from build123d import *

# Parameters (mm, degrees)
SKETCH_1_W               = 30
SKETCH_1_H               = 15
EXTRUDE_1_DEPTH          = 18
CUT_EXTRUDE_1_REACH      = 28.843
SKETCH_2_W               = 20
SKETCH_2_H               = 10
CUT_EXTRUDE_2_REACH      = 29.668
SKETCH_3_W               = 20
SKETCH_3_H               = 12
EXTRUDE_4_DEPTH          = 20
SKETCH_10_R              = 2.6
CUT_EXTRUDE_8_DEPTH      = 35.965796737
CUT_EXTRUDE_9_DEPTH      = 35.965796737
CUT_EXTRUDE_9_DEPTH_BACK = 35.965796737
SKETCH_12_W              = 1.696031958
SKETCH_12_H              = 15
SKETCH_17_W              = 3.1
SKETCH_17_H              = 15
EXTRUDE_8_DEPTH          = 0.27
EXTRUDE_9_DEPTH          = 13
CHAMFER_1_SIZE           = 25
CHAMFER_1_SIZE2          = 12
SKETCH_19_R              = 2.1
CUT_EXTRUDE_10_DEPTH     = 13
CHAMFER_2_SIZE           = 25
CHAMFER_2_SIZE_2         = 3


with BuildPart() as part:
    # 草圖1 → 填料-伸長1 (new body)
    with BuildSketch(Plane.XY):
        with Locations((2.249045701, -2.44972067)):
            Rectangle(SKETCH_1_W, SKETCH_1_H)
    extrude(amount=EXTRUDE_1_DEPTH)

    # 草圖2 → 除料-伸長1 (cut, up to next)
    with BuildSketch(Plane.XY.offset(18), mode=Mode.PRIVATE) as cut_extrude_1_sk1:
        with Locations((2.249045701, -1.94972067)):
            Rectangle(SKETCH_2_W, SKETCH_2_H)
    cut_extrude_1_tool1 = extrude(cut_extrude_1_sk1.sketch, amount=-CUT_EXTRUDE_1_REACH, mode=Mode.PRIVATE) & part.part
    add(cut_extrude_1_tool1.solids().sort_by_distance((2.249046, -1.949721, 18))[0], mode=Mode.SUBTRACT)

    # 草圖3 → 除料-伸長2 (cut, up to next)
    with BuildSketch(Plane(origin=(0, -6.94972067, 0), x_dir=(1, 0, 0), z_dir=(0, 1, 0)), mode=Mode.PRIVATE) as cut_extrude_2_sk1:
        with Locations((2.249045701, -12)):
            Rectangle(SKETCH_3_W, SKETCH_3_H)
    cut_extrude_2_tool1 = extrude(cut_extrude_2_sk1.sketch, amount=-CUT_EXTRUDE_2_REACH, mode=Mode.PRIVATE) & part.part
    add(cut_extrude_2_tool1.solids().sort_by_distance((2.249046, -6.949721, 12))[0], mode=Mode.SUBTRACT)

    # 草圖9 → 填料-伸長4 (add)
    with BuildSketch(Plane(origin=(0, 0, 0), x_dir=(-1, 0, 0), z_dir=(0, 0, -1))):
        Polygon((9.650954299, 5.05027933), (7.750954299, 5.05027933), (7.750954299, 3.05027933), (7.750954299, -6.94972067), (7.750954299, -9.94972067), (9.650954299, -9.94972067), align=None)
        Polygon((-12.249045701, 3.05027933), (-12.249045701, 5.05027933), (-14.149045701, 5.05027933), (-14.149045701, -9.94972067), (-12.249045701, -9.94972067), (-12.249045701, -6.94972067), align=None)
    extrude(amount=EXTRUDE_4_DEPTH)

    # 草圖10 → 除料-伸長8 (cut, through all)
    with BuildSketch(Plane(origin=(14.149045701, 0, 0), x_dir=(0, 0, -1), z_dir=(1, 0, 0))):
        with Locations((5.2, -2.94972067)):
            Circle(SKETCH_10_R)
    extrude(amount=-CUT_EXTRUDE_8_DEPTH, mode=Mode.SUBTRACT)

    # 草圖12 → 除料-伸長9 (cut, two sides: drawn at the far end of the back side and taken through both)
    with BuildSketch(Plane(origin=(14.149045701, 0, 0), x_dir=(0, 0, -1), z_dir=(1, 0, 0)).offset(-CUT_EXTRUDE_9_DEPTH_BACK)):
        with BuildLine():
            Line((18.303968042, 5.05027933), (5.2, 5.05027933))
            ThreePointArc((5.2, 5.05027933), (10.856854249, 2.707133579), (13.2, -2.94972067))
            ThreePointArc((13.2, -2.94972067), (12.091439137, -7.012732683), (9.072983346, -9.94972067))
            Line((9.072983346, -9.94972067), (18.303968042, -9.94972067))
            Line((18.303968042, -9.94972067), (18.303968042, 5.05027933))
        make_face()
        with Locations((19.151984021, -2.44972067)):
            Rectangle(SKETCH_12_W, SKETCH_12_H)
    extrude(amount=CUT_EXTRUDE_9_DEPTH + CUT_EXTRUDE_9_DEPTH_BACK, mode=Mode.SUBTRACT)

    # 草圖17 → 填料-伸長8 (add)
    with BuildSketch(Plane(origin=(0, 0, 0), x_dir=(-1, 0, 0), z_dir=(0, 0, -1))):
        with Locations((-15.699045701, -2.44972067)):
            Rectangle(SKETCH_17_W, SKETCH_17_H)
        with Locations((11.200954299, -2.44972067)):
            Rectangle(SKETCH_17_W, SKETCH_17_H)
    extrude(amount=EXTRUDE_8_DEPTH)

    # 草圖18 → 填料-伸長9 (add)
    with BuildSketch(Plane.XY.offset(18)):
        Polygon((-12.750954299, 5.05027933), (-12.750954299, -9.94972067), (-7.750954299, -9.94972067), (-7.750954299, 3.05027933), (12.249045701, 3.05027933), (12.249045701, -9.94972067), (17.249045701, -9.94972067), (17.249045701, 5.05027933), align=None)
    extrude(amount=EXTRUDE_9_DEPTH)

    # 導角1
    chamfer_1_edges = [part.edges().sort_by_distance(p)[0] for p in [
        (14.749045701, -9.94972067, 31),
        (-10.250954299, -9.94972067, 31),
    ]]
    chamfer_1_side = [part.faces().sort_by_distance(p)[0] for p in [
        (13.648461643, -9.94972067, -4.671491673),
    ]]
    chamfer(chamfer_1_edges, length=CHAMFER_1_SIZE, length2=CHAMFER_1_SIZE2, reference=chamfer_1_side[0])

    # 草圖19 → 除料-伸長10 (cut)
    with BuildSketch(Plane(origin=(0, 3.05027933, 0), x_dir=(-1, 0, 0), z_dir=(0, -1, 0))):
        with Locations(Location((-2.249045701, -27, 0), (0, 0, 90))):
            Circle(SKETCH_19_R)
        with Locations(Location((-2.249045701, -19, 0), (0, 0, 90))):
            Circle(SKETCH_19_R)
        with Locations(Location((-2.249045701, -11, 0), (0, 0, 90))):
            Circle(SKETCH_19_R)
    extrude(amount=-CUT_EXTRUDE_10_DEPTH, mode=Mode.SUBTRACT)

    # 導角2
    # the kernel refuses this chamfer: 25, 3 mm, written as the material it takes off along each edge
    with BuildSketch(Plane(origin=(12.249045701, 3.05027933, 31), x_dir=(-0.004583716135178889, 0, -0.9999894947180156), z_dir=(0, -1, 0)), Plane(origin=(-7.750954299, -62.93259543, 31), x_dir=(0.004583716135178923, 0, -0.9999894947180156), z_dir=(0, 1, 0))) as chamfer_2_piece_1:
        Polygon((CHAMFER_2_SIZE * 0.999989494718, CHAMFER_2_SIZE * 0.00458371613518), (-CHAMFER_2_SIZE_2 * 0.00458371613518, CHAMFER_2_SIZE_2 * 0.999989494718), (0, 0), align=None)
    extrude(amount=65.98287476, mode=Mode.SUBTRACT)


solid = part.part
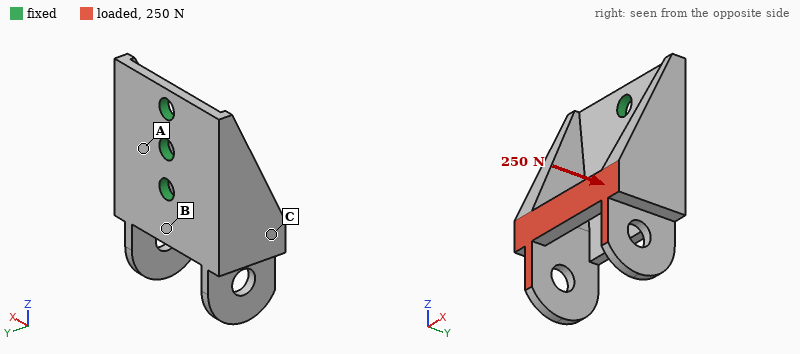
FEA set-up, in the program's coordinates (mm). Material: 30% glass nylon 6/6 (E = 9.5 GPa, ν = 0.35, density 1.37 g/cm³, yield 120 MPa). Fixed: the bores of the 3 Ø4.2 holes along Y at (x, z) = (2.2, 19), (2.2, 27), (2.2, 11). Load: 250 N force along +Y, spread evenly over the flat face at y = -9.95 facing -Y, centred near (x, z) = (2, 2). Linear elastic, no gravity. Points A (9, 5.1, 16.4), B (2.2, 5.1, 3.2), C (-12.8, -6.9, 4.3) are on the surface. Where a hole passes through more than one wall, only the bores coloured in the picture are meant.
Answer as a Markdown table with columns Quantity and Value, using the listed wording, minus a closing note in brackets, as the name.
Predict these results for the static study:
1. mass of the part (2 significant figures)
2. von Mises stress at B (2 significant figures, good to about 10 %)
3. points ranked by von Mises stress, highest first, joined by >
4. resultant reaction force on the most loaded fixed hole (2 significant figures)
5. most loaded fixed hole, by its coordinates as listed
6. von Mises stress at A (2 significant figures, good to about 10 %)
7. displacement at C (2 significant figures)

| Quantity | Value |
|---|---|
| mass of the part | 6.7 g |
| von Mises stress at B | 46 MPa |
| points ranked by von Mises stress, highest first, joined by > | B > A > C |
| resultant reaction force on the most loaded fixed hole | 330 N |
| most loaded fixed hole, by its coordinates as listed | (2.2, 11) |
| von Mises stress at A | 25 MPa |
| displacement at C | 0.31 mm |
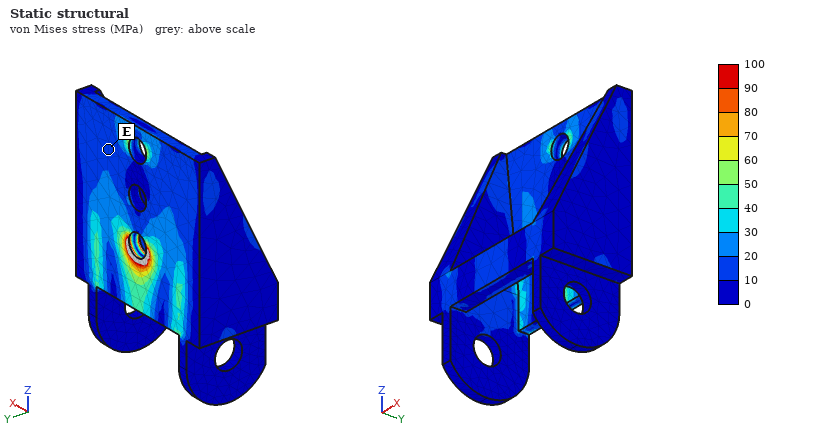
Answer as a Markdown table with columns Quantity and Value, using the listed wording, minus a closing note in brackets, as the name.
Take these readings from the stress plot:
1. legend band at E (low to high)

| Quantity | Value |
|---|---|
| legend band at E | 10 to 20 MPa |
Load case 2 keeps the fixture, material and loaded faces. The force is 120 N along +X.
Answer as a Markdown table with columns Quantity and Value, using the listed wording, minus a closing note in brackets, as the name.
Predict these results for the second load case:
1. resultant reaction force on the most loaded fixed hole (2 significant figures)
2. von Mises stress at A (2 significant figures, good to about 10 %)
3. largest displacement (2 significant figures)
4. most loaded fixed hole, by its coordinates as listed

| Quantity | Value |
|---|---|
| resultant reaction force on the most loaded fixed hole | 150 N |
| von Mises stress at A | 27 MPa |
| largest displacement | 0.57 mm |
| most loaded fixed hole, by its coordinates as listed | (2.2, 11) |
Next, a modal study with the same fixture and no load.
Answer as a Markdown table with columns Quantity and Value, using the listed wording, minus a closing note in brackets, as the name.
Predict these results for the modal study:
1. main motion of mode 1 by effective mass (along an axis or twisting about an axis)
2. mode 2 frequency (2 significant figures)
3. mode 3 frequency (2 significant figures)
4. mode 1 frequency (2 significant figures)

| Quantity | Value |
|---|---|
| main motion of mode 1 by effective mass | along X |
| mode 2 frequency | 2000 Hz |
| mode 3 frequency | 3500 Hz |
| mode 1 frequency | 1400 Hz |
